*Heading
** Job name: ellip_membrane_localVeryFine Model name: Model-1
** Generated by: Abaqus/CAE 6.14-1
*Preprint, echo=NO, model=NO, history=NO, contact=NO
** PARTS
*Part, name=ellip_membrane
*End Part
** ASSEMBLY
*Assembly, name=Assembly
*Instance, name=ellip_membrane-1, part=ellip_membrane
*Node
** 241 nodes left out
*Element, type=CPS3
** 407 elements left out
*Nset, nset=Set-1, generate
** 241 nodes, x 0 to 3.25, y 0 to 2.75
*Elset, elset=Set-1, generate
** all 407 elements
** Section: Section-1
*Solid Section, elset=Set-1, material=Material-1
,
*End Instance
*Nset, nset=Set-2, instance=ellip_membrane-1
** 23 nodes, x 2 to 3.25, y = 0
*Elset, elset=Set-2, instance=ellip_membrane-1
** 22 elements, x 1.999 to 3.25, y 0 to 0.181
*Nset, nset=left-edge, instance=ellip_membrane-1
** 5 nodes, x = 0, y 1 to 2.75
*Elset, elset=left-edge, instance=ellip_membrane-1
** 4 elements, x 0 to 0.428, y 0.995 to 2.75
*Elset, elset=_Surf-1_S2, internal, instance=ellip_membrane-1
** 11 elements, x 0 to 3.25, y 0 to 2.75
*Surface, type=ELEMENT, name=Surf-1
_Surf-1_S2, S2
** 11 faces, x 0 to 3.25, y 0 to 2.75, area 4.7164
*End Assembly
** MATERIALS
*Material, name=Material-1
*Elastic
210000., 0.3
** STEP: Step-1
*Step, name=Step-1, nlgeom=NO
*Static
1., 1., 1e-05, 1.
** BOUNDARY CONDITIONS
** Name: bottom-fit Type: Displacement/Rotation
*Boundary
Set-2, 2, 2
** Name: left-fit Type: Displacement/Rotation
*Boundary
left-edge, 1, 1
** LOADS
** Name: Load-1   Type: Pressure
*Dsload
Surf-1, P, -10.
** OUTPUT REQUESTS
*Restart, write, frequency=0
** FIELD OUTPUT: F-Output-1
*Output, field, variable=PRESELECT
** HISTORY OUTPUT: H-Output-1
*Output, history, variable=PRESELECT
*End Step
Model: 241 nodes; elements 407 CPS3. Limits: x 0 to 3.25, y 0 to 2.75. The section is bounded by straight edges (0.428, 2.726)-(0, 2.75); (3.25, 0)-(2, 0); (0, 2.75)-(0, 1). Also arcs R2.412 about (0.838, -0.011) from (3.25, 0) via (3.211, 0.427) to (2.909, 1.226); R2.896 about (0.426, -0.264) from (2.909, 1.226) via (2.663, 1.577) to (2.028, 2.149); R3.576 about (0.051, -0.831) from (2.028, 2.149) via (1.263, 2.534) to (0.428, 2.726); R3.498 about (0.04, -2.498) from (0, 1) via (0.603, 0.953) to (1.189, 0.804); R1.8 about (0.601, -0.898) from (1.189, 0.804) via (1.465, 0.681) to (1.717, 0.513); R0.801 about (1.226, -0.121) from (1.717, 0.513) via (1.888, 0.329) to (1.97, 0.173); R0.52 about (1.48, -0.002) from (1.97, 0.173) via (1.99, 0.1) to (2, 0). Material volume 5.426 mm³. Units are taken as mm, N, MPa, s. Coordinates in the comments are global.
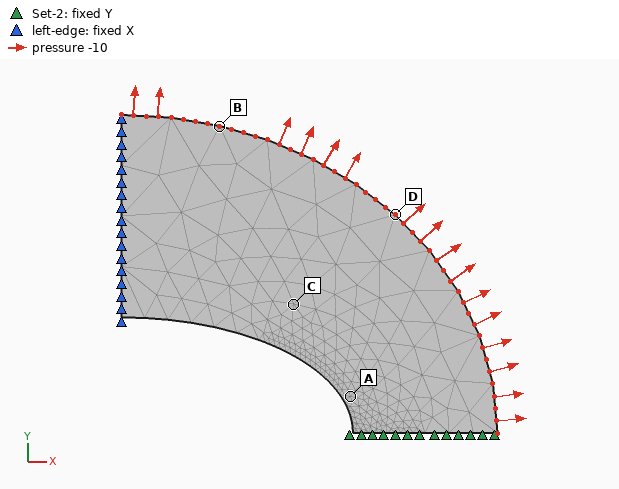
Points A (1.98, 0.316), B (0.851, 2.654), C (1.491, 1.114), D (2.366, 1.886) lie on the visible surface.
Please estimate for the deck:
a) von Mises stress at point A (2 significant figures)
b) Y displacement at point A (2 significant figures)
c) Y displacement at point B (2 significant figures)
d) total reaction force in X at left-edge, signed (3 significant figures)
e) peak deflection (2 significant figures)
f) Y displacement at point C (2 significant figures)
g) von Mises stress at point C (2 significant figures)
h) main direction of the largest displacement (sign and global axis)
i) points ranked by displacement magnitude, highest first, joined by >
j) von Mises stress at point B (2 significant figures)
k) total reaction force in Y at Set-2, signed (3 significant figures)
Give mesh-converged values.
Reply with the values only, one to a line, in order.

54 MPa
1.1e-04 mm
4.9e-04 mm
-27.5 N
5.5e-04 mm
3.4e-04 mm
20 MPa
+Y
B > C > D > A
26 MPa
-32.5 N
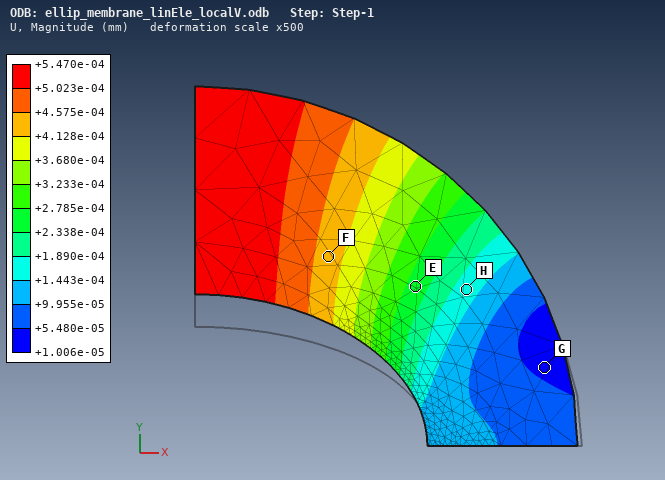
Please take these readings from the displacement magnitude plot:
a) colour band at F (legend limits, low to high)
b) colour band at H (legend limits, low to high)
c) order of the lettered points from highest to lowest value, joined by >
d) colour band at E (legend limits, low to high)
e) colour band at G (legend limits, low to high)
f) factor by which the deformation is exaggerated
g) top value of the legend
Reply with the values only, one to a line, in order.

+4.128e-04 to +4.575e-04 mm
+1.443e-04 to +1.890e-04 mm
F > E > H > G
+2.338e-04 to +2.785e-04 mm
+1.006e-05 to +5.480e-05 mm
500
+5.470e-04 mm
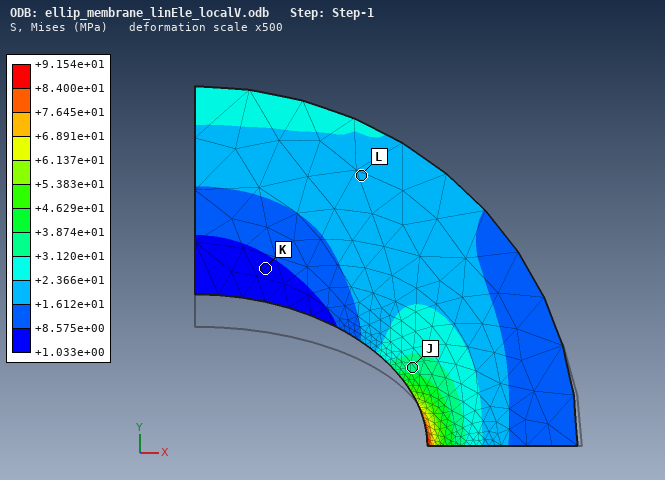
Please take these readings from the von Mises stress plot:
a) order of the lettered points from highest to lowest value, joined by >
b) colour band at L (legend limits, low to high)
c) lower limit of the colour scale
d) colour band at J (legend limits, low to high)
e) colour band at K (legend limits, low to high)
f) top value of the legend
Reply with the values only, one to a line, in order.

J > L > K
+1.612e+01 to +2.366e+01 MPa
+1.033e+00 MPa
+3.120e+01 to +3.874e+01 MPa
+1.033e+00 to +8.575e+00 MPa
+9.154e+01 MPa
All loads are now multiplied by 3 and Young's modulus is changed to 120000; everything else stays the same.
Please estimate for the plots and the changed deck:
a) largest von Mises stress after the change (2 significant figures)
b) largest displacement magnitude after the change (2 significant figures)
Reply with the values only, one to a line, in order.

270 MPa
0.0029 mm
